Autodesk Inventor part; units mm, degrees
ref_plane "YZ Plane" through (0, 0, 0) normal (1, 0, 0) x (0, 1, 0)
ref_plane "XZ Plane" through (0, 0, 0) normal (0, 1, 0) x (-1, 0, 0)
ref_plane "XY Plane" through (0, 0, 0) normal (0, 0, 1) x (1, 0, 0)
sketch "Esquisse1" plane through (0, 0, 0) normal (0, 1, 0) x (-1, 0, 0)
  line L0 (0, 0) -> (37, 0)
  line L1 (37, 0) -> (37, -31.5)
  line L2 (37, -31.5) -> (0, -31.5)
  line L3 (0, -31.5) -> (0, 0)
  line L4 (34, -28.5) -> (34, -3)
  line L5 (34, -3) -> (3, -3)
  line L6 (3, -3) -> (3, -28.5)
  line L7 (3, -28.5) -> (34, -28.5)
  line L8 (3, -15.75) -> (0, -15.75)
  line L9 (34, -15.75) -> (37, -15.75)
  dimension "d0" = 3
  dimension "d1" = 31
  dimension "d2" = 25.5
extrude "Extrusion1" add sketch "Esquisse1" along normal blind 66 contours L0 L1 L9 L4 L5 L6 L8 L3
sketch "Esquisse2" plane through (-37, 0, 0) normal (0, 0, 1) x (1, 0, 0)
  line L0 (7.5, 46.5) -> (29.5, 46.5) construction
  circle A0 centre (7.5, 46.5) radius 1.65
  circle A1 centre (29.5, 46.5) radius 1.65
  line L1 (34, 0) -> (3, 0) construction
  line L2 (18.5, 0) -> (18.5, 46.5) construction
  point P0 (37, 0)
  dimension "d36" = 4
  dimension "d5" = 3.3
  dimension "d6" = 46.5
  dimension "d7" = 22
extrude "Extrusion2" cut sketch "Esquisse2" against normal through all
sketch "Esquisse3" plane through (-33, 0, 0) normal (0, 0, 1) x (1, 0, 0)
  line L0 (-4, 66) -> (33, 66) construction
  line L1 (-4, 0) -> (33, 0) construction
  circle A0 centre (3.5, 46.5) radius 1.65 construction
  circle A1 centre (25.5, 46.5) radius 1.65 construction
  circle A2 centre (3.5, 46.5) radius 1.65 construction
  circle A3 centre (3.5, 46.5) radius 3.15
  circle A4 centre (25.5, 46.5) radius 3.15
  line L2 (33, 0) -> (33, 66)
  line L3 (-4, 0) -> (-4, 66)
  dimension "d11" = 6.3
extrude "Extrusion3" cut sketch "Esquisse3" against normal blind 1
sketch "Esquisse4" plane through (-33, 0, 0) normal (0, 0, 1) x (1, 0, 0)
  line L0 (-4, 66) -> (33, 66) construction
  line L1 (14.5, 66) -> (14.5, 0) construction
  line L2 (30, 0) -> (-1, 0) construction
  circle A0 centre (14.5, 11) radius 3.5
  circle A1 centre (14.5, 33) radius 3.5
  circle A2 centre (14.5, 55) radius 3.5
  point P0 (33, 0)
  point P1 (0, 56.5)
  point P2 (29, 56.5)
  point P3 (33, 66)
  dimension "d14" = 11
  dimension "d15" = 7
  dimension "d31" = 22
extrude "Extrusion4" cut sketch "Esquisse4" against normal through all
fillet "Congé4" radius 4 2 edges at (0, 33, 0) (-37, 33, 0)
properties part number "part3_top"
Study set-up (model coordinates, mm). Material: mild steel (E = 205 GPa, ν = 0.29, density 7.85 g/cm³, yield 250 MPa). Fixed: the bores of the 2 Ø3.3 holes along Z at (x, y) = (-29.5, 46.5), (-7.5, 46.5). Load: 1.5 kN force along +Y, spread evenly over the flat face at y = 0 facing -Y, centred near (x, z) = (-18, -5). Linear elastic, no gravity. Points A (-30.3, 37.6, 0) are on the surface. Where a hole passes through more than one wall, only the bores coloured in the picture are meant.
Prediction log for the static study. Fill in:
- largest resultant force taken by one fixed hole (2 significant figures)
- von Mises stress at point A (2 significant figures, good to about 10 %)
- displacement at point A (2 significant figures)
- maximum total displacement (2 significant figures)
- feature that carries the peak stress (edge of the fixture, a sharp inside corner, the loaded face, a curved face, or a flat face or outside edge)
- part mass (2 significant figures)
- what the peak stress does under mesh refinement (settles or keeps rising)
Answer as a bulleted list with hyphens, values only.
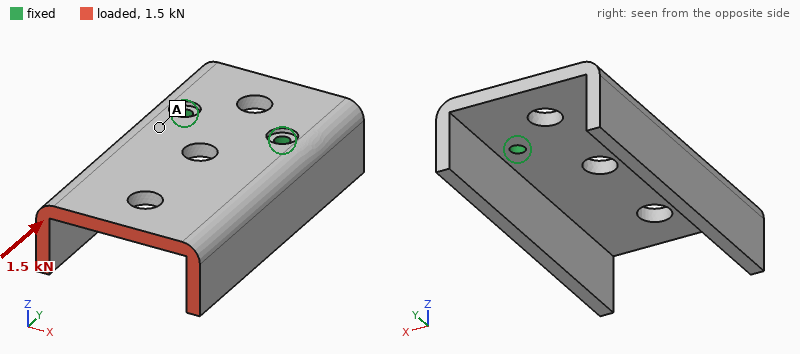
- 750 N
- 17 MPa
- 9.4 µm
- 63 µm
- edge of the fixture
- 90 g
- keeps rising
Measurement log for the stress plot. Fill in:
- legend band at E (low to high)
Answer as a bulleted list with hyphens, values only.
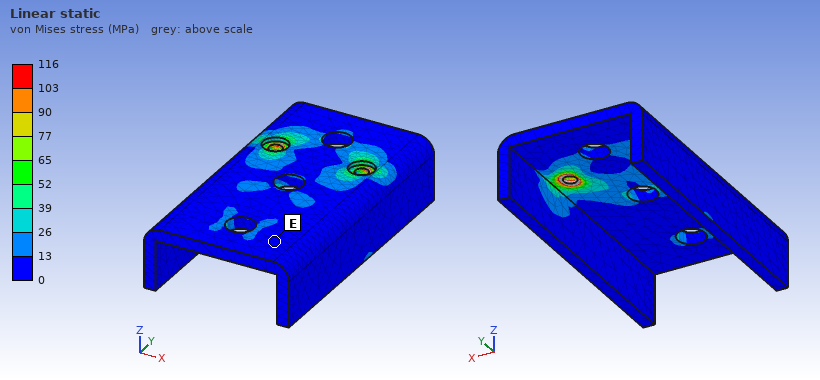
- 0 to 13 MPa
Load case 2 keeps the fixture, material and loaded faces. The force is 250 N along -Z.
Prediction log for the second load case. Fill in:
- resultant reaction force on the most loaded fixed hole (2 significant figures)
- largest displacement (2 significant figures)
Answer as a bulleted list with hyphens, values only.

- 130 N
- 0.17 mm
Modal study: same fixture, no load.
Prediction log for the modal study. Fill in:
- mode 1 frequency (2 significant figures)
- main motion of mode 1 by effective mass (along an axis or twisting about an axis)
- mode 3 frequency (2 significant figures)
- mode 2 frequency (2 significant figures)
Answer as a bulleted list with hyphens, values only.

- 1300 Hz
- along Z
- 4900 Hz
- 2300 Hz
